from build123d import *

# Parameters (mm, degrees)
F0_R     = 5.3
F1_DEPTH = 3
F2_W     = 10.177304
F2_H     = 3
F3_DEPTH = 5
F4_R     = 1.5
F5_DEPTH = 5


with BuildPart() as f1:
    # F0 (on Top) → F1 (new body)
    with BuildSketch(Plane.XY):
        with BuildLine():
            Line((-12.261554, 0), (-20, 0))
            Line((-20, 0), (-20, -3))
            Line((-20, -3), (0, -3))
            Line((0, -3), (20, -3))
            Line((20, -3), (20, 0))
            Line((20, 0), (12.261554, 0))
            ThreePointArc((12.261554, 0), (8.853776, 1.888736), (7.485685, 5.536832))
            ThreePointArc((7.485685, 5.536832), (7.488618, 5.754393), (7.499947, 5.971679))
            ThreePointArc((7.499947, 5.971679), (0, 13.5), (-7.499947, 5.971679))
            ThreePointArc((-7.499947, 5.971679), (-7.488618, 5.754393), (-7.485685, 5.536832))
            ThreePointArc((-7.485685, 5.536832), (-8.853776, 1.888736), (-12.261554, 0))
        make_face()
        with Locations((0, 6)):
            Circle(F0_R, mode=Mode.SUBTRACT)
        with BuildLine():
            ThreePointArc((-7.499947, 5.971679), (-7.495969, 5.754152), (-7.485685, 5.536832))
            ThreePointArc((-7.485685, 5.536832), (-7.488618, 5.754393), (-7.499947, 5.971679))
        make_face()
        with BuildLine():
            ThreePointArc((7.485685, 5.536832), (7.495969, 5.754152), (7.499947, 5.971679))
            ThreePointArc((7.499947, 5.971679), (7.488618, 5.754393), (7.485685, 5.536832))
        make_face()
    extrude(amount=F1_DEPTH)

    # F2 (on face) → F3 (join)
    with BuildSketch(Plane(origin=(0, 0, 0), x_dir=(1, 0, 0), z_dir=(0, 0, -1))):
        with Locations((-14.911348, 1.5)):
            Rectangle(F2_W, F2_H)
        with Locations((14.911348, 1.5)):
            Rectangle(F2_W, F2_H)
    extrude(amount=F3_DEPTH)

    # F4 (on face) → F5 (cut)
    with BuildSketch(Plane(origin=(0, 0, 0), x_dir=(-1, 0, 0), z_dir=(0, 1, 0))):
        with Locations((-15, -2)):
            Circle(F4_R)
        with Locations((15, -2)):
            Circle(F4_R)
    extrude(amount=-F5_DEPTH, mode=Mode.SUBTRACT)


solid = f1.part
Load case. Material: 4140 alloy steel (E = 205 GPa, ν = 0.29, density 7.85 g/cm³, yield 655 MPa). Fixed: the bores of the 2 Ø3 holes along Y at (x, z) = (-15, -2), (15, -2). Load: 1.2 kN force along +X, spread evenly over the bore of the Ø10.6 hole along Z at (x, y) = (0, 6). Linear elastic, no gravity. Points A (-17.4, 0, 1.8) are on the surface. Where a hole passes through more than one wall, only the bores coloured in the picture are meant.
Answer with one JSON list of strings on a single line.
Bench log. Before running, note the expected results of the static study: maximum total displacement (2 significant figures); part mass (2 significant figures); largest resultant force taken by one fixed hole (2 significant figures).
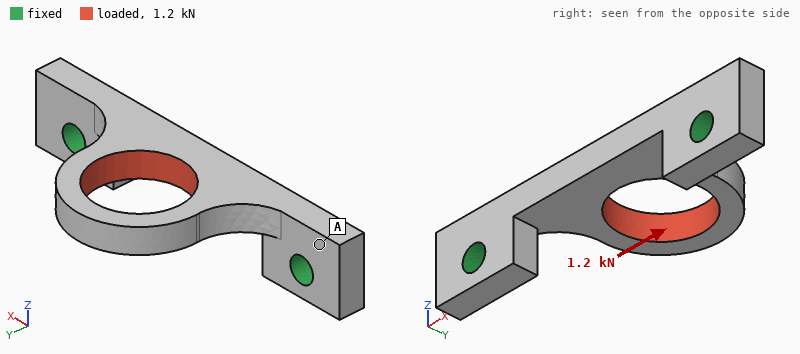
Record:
["35 µm", "7.3 g", "700 N"]
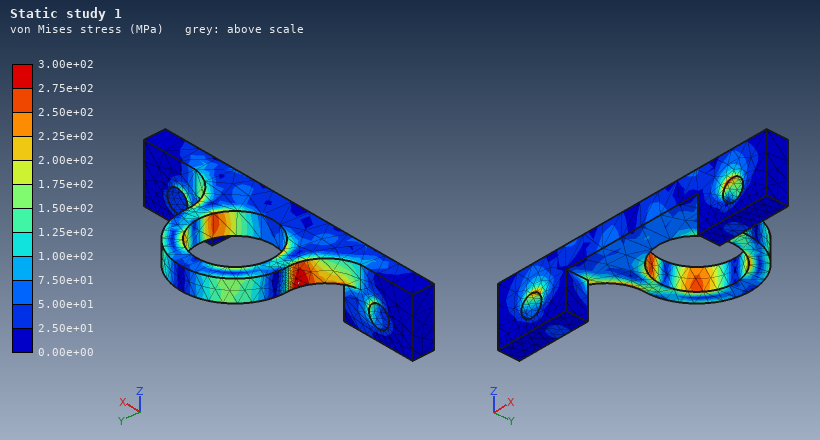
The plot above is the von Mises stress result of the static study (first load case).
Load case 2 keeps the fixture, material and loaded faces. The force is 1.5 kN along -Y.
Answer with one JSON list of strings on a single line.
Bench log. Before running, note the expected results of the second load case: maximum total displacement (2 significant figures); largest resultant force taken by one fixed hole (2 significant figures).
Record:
["43 µm", "830 N"]
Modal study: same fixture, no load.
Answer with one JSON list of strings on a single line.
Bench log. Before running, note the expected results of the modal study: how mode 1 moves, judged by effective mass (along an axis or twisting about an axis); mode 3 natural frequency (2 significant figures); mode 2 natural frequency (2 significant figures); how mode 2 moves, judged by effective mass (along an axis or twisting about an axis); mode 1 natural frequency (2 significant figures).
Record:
["along Z", "21 kHz", "19 kHz", "along Y", "7700 Hz"]
